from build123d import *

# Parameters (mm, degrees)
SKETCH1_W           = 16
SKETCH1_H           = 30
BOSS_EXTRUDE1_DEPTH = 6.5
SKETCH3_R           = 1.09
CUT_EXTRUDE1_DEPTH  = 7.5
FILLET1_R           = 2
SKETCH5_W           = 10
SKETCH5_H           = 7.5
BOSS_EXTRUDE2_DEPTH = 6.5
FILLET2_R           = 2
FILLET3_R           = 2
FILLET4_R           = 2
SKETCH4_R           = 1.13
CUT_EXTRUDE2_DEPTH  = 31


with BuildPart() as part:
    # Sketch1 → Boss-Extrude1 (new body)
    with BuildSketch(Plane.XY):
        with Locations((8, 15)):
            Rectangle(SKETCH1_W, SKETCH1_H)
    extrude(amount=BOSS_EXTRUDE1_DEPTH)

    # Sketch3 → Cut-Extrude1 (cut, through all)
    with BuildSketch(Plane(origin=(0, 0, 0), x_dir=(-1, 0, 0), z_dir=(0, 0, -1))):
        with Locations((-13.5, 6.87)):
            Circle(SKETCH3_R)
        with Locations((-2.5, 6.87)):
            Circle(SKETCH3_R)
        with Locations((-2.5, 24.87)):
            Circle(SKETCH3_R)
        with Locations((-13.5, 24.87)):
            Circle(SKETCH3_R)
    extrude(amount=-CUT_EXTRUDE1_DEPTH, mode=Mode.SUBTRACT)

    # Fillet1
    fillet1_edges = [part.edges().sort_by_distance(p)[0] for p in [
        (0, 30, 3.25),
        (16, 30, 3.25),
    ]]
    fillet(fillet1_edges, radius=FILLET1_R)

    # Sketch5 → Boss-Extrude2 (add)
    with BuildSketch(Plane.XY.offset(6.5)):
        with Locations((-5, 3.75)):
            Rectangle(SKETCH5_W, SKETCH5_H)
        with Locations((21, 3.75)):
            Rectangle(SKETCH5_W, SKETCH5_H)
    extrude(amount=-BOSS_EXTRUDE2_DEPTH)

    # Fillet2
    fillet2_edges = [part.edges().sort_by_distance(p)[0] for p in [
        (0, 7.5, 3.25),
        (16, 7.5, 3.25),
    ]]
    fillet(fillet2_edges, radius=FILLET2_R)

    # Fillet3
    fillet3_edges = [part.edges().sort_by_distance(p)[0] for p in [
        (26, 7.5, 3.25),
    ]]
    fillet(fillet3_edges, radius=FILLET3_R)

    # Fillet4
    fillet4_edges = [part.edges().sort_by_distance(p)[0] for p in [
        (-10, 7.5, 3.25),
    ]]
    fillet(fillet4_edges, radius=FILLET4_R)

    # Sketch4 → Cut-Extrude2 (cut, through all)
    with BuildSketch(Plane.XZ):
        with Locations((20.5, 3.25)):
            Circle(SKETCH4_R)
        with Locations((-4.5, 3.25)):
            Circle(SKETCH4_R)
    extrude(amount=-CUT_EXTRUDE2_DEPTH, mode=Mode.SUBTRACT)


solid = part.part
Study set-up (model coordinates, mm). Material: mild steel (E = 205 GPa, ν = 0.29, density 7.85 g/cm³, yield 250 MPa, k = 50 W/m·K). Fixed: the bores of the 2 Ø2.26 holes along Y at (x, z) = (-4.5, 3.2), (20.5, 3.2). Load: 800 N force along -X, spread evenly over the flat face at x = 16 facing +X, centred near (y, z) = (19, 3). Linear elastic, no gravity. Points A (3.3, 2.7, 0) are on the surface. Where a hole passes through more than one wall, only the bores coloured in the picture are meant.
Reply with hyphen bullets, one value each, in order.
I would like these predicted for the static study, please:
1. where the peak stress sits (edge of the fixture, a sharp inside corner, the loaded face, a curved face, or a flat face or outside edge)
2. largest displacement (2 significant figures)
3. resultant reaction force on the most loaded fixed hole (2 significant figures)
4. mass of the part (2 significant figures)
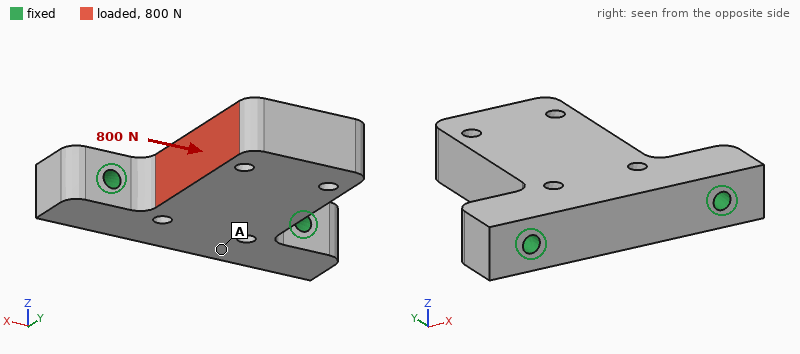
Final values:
- a curved face
- 7.0 µm
- 680 N
- 31 g
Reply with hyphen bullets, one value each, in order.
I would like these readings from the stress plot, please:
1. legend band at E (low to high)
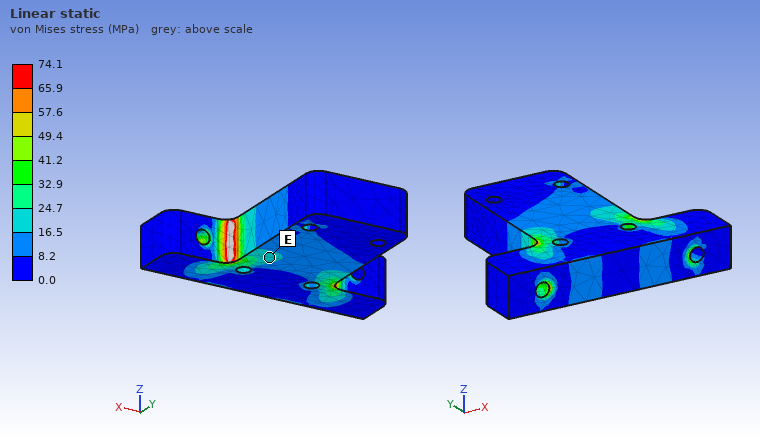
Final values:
- 16.5 to 24.7 MPa
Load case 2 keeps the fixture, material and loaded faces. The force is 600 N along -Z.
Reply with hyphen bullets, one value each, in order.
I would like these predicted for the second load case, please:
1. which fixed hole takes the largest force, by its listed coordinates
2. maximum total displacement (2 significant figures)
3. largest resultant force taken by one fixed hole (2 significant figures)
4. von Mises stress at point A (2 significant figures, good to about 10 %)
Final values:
- (20.5, 3.2)
- 50 µm
- 530 N
- 50 MPa
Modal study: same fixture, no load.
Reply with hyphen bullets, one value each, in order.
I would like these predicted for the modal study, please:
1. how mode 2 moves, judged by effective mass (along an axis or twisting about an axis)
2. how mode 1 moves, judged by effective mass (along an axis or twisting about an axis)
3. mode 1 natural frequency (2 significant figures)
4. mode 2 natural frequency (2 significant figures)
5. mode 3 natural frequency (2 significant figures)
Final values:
- along X
- along Z
- 5300 Hz
- 15 kHz
- 21 kHz
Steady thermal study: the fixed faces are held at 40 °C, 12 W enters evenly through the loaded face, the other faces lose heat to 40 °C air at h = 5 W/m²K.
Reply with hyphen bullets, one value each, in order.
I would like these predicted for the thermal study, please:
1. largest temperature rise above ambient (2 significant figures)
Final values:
- 56 K
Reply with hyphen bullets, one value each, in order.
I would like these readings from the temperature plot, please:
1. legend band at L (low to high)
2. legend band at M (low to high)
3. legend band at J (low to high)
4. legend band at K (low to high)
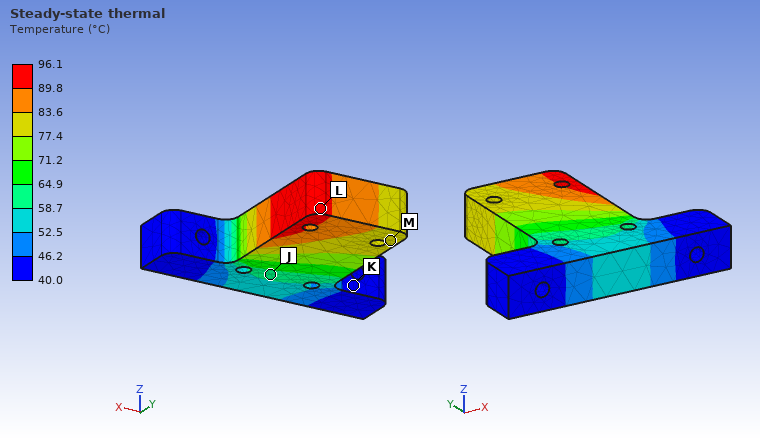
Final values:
- 89.8 to 96.1 °C
- 77.4 to 83.6 °C
- 58.7 to 64.9 °C
- 40.0 to 46.2 °C
